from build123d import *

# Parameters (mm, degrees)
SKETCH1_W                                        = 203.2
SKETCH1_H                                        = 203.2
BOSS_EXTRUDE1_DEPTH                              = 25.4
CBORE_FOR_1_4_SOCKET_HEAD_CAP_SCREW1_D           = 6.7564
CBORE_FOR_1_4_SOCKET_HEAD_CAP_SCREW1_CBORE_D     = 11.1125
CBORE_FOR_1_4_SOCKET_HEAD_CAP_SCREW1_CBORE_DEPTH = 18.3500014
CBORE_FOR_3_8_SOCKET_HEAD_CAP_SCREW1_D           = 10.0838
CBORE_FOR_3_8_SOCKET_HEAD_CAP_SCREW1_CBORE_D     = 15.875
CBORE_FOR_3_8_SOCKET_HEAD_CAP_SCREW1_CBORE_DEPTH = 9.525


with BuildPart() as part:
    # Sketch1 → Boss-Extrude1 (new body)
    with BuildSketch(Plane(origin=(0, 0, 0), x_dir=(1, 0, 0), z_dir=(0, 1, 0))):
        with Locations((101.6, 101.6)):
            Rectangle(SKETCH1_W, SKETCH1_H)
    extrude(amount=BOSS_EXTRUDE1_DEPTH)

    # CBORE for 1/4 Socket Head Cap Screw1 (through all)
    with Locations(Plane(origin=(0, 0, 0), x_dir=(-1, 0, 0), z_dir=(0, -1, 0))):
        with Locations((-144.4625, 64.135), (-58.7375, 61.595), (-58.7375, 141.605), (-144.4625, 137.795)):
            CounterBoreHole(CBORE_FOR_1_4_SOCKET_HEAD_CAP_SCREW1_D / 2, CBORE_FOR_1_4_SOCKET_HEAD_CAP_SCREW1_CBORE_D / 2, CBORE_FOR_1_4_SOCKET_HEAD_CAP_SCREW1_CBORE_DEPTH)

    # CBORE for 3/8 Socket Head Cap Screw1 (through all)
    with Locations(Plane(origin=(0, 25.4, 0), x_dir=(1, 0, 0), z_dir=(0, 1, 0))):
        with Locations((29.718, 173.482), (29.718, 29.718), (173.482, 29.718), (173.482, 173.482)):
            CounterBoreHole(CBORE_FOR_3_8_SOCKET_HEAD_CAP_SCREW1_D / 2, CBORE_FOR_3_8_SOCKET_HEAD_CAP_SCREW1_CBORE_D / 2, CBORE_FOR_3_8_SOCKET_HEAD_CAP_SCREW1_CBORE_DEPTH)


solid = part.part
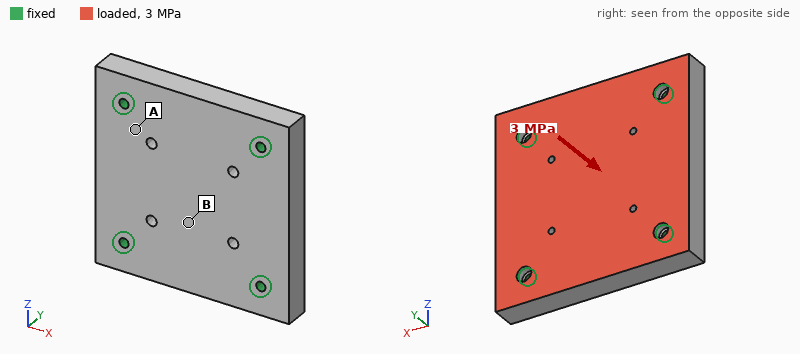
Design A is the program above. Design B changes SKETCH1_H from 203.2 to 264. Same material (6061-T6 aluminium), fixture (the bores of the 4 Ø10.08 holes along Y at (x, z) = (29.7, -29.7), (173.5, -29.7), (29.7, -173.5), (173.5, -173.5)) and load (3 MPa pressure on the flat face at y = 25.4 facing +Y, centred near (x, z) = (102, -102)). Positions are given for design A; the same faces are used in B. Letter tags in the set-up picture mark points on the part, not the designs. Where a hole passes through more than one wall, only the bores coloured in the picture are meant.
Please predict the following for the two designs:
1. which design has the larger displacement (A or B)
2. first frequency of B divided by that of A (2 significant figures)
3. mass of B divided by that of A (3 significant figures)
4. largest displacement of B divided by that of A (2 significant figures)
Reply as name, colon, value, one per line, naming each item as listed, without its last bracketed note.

which design has the larger displacement: B
first frequency of B divided by that of A: 0.85
mass of B divided by that of A: 1.31
largest displacement of B divided by that of A: 1.3
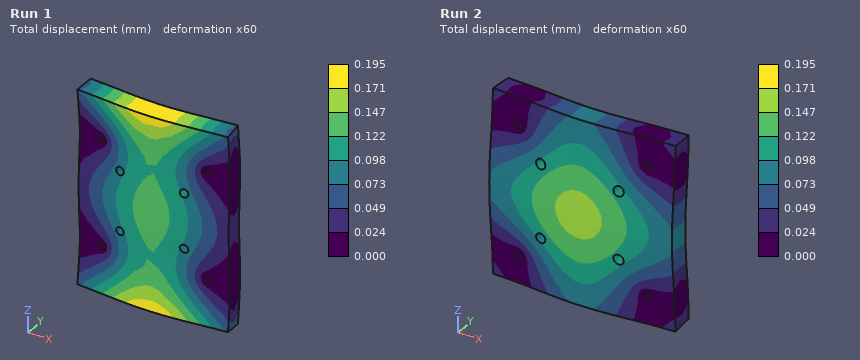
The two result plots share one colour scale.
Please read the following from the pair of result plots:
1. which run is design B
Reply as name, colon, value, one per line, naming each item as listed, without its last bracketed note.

which run is design B: Run 1
